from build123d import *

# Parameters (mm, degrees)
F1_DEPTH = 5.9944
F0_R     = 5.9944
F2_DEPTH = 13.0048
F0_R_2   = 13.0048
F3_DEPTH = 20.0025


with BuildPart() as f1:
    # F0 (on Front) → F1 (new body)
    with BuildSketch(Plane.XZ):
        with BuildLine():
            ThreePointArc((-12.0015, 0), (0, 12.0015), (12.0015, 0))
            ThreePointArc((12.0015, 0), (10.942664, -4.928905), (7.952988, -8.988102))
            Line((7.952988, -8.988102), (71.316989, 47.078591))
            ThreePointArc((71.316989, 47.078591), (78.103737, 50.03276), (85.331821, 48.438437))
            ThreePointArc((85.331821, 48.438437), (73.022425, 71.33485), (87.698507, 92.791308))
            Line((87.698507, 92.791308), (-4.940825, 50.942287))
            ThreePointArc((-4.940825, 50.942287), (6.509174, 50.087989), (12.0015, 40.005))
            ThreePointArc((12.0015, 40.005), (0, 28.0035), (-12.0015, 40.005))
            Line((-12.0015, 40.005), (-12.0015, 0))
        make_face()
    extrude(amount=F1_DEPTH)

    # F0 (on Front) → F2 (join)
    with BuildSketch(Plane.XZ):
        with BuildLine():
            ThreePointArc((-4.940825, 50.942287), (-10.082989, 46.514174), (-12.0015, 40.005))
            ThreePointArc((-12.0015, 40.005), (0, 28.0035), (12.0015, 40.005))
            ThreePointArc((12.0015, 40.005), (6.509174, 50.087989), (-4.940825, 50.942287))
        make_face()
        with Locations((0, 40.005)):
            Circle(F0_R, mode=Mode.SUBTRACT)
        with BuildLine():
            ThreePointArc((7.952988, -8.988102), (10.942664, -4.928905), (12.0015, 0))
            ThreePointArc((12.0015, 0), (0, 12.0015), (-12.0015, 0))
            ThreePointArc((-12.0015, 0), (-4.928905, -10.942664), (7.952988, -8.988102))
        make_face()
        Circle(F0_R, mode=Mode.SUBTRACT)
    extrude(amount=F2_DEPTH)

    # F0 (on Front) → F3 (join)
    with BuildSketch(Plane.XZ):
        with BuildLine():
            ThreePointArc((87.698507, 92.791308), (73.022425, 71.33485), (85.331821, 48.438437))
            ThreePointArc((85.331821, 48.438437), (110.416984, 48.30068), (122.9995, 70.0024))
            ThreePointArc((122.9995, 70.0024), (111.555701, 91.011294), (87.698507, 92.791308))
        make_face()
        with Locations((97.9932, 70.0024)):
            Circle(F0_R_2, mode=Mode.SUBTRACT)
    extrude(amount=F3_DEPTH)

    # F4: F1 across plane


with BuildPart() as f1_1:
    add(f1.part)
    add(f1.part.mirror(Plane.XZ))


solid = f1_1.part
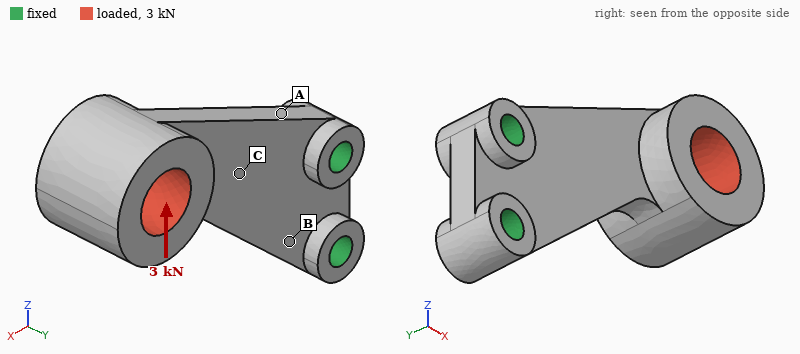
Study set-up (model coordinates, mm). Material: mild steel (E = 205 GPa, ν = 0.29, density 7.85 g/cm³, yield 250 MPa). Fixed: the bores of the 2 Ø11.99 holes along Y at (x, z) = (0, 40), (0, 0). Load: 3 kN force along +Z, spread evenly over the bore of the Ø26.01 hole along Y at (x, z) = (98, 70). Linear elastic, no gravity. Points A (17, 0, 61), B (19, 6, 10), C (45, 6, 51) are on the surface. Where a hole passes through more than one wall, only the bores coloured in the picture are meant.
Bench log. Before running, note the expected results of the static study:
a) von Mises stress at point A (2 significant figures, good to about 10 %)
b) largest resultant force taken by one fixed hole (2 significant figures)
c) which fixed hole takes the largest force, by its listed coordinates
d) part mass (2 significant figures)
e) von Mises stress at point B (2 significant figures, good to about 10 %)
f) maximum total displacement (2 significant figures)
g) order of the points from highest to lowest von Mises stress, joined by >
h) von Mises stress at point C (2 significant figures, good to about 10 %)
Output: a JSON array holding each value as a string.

["45 MPa", "7.1 kN", "(0, 0)", "950 g", "33 MPa", "83 µm", "A > B > C", "7.8 MPa"]
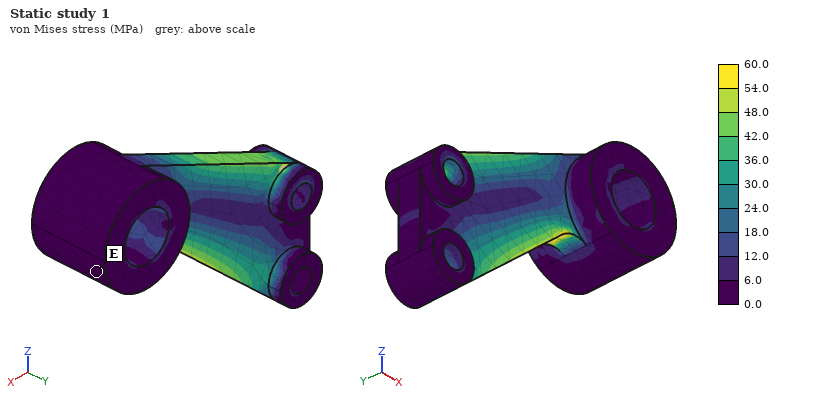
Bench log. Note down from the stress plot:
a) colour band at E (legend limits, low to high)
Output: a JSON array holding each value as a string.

["0.0 to 6.0 MPa"]
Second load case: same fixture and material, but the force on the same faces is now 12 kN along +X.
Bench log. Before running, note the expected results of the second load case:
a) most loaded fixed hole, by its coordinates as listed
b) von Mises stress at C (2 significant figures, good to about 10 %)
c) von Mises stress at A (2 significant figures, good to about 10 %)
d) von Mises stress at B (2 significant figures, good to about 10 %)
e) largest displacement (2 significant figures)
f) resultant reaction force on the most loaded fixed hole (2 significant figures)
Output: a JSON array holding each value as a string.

["(0, 40)", "33 MPa", "97 MPa", "40 MPa", "0.12 mm", "19 kN"]
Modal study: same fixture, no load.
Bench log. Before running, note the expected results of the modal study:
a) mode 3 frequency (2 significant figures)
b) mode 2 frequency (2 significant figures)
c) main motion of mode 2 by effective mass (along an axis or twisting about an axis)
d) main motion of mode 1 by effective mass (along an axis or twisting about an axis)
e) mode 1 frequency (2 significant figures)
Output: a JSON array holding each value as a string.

["1900 Hz", "1500 Hz", "along Z", "along Y", "460 Hz"]
